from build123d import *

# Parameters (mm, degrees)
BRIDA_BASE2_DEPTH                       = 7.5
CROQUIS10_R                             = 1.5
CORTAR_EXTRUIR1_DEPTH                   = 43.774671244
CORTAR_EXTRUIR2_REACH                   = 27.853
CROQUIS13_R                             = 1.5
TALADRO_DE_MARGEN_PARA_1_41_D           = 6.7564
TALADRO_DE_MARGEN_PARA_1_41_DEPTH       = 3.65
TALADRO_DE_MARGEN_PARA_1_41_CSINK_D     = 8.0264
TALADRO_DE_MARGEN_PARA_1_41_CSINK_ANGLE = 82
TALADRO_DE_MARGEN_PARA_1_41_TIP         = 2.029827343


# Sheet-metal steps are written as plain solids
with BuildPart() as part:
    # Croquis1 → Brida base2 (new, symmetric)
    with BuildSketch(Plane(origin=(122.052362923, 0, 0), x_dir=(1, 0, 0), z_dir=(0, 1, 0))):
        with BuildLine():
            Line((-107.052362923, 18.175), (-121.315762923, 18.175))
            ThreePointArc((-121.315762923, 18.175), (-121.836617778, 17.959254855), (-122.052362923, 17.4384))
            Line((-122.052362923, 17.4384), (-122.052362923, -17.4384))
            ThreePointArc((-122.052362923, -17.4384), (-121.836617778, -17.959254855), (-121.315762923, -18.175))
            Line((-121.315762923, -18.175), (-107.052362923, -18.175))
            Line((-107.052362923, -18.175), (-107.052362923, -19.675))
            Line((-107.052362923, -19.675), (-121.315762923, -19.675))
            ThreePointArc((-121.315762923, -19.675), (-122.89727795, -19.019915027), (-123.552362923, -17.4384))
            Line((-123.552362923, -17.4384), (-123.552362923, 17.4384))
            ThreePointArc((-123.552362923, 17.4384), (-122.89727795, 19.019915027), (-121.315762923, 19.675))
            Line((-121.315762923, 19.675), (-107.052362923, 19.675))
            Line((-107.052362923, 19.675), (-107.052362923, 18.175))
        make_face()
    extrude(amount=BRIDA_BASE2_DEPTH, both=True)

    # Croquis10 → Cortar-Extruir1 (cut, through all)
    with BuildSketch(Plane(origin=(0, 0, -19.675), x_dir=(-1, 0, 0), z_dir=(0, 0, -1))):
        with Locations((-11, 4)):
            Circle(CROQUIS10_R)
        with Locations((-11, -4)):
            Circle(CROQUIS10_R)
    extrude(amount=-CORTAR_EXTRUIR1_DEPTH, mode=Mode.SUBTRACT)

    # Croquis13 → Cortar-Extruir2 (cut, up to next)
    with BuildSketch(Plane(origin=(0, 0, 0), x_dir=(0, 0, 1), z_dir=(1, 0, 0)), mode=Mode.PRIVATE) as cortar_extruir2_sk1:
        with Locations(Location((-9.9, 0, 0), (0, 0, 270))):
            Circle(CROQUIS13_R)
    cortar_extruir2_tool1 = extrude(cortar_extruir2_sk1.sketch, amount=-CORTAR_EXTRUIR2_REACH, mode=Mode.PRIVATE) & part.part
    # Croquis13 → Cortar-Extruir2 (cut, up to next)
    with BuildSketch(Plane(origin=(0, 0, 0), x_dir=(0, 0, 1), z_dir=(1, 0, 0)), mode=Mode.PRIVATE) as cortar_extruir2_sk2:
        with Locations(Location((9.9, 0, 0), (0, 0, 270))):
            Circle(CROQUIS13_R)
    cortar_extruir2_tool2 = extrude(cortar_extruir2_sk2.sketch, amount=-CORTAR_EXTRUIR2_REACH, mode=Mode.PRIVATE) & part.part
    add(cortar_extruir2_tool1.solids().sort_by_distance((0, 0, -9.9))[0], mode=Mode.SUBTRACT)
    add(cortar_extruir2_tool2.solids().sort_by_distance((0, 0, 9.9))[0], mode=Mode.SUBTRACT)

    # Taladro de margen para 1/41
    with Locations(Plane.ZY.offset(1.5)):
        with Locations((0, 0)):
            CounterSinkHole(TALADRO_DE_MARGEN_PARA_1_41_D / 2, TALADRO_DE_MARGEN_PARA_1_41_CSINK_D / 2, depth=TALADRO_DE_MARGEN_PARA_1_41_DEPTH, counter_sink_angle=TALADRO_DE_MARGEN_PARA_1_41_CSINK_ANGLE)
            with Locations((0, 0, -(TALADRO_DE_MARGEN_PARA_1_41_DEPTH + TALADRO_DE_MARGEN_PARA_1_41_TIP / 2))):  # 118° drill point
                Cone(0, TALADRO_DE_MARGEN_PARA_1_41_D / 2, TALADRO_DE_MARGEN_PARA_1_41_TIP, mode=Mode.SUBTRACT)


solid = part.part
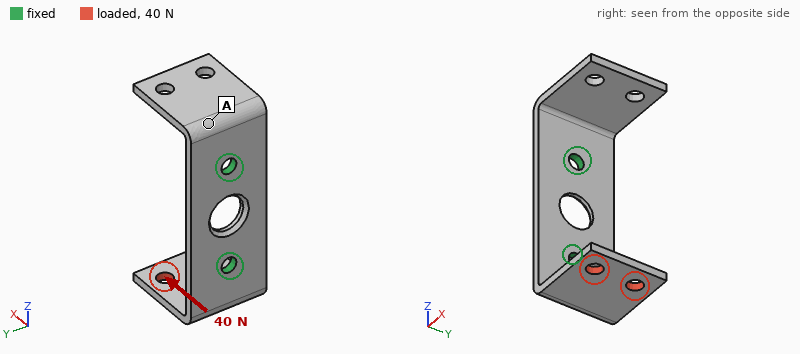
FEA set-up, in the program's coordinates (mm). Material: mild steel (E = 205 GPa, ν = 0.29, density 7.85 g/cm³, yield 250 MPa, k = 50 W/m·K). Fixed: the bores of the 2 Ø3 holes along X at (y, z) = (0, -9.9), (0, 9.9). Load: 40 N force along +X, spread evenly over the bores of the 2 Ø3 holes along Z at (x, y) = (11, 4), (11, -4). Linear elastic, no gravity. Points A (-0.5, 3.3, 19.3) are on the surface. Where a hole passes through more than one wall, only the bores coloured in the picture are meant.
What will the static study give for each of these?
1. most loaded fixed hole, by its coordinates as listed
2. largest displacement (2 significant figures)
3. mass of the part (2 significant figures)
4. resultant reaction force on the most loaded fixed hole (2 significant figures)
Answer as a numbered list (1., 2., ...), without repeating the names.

1. (0, -9.9)
2. 29 µm
3. 11 g
4. 42 N
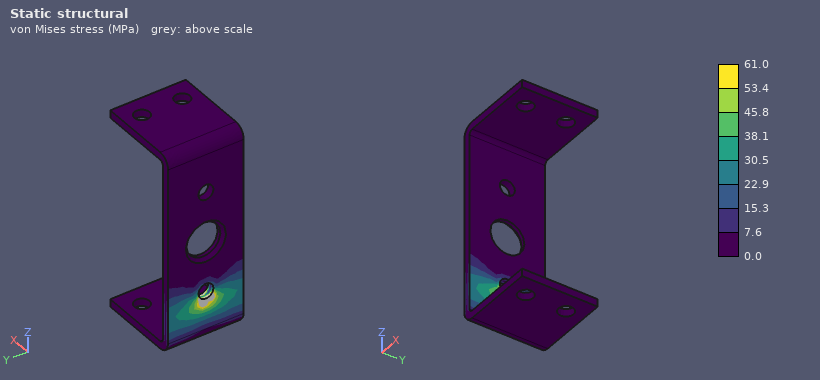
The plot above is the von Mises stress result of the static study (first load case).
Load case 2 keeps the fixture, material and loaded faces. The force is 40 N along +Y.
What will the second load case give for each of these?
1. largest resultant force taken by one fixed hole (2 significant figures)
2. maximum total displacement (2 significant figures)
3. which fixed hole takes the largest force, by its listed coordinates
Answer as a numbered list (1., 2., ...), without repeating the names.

1. 50 N
2. 44 µm
3. (0, -9.9)
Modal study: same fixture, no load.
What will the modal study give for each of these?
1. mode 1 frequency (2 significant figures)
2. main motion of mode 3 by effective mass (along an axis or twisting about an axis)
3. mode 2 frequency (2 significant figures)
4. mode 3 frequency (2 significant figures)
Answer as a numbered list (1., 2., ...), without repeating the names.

1. 2800 Hz
2. twisting about X
3. 2800 Hz
4. 4200 Hz
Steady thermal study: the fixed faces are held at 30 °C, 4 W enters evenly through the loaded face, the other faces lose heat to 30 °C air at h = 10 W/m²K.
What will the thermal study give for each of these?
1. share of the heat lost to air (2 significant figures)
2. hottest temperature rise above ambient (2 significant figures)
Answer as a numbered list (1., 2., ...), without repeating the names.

1. 8.6 %
2. 76 K
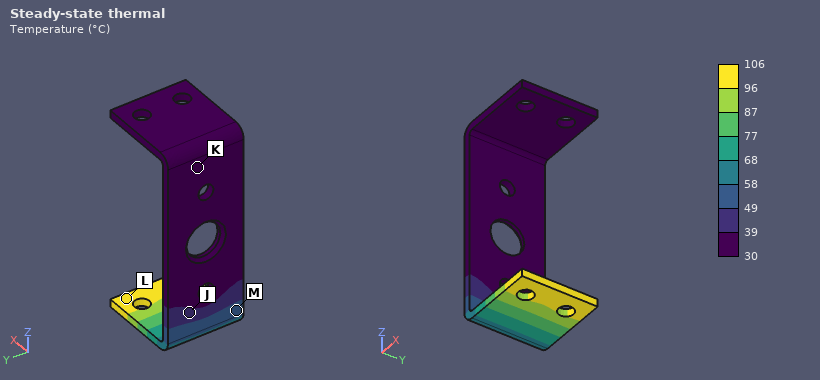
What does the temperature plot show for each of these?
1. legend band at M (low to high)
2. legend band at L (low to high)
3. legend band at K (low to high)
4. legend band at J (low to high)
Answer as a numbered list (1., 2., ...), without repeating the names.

1. 49 to 58 °C
2. 96 to 106 °C
3. 30 to 39 °C
4. 39 to 49 °C
